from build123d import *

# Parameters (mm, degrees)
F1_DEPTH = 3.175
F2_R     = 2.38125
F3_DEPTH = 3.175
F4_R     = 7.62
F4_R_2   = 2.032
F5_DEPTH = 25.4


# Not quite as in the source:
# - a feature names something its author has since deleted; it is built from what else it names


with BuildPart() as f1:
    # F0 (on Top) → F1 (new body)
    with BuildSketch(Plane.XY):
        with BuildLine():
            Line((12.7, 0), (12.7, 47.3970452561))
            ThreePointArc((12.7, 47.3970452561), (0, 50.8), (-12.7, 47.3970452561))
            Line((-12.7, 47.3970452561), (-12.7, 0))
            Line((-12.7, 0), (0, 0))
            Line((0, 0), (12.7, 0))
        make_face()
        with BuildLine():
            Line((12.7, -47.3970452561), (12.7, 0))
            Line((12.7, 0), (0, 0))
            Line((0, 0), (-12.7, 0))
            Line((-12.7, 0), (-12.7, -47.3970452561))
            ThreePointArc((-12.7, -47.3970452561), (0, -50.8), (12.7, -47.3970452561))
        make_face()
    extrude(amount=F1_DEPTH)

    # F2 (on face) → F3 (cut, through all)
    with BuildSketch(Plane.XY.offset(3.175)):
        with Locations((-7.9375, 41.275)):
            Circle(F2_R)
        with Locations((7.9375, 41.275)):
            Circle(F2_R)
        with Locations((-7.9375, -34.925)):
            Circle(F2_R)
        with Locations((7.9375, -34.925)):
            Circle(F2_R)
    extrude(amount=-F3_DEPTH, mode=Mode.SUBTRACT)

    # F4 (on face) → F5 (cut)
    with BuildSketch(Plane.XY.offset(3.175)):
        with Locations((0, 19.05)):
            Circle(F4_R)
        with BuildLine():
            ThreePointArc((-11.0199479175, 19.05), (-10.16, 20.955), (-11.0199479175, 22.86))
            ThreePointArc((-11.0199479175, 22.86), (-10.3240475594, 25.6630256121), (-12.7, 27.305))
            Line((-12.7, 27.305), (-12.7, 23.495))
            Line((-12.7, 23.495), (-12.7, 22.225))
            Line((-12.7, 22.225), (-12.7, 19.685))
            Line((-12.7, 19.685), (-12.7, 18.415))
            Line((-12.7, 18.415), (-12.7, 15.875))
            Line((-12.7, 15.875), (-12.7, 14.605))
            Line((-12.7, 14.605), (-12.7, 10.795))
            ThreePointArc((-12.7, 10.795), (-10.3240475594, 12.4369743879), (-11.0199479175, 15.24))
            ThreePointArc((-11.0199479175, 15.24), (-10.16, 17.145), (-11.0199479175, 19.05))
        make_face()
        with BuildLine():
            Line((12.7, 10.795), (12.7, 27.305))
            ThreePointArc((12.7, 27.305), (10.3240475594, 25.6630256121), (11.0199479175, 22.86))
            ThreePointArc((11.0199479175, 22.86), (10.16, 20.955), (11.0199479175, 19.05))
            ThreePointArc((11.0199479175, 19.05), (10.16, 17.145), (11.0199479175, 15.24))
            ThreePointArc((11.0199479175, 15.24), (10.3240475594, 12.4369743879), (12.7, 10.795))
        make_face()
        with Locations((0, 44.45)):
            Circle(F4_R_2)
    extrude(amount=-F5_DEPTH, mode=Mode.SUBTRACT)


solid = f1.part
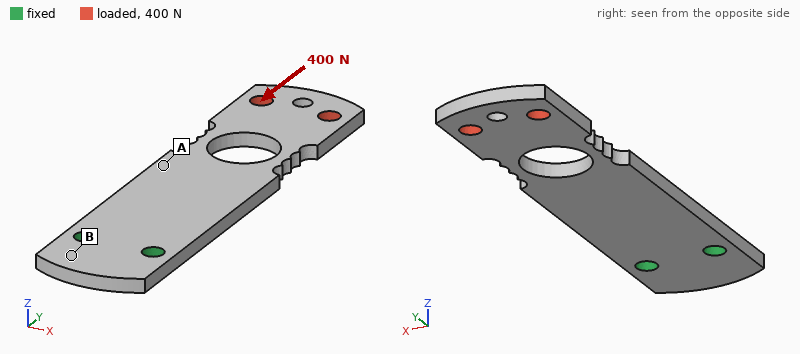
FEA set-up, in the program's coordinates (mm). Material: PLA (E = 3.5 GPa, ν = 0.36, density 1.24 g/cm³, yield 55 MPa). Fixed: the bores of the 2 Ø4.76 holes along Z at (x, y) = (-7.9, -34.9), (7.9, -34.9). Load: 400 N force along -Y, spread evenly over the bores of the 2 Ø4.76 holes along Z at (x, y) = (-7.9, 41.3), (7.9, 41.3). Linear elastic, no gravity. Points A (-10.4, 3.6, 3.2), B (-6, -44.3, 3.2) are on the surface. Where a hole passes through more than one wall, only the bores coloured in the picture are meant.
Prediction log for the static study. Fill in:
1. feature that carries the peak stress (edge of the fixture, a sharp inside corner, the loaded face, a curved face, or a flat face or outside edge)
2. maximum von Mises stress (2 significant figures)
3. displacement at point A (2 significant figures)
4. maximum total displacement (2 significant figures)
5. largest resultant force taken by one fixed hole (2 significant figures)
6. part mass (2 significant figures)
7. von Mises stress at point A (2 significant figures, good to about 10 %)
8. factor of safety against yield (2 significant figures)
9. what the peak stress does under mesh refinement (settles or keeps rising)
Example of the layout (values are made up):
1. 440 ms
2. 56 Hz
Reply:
1. a curved face
2. 44 MPa
3. 0.057 mm
4. 0.20 mm
5. 200 N
6. 8.6 g
7. 6.8 MPa
8. 1.2
9. settles
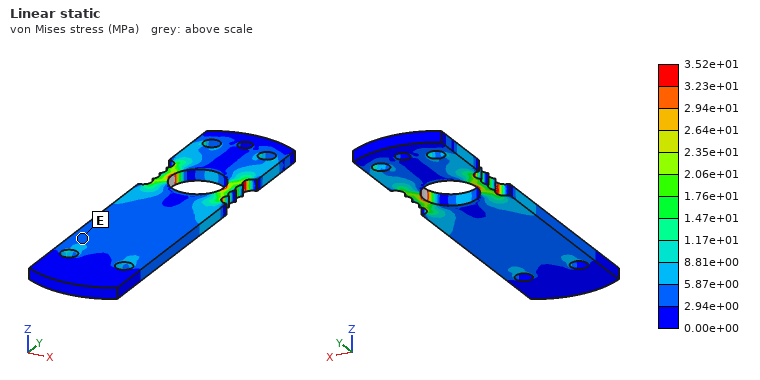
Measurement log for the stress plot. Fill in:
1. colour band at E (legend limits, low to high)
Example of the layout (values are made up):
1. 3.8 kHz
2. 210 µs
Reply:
1. 2.94e+00 to 5.87e+00 MPa
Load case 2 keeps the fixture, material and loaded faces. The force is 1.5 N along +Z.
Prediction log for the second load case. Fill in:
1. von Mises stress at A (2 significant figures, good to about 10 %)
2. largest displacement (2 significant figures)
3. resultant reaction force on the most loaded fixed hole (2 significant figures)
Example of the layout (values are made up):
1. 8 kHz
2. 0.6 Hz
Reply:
1. 1.4 MPa
2. 1.2 mm
3. 0.75 N
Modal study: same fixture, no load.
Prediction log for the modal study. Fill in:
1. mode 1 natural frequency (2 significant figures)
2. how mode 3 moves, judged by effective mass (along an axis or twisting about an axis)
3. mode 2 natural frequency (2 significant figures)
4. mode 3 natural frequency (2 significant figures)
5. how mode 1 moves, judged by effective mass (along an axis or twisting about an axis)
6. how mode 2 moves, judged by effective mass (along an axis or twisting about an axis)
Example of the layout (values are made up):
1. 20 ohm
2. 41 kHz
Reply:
1. 130 Hz
2. twisting about Y
3. 660 Hz
4. 780 Hz
5. along Z
6. along Z
